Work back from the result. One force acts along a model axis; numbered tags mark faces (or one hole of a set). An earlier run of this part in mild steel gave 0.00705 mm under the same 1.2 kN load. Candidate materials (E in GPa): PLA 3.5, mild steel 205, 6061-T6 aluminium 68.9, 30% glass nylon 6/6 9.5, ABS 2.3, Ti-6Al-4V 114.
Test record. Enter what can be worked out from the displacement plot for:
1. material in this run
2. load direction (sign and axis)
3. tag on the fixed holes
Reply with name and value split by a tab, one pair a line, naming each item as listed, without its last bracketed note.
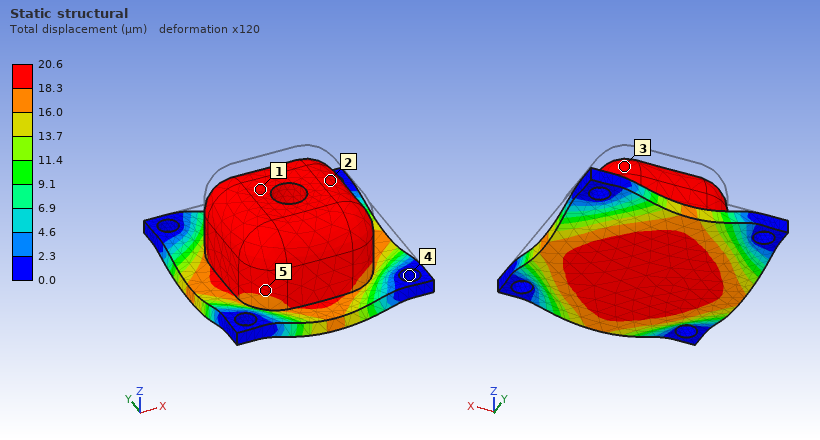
material in this run	6061-T6 aluminium
load direction	-Z
tag on the fixed holes	4
